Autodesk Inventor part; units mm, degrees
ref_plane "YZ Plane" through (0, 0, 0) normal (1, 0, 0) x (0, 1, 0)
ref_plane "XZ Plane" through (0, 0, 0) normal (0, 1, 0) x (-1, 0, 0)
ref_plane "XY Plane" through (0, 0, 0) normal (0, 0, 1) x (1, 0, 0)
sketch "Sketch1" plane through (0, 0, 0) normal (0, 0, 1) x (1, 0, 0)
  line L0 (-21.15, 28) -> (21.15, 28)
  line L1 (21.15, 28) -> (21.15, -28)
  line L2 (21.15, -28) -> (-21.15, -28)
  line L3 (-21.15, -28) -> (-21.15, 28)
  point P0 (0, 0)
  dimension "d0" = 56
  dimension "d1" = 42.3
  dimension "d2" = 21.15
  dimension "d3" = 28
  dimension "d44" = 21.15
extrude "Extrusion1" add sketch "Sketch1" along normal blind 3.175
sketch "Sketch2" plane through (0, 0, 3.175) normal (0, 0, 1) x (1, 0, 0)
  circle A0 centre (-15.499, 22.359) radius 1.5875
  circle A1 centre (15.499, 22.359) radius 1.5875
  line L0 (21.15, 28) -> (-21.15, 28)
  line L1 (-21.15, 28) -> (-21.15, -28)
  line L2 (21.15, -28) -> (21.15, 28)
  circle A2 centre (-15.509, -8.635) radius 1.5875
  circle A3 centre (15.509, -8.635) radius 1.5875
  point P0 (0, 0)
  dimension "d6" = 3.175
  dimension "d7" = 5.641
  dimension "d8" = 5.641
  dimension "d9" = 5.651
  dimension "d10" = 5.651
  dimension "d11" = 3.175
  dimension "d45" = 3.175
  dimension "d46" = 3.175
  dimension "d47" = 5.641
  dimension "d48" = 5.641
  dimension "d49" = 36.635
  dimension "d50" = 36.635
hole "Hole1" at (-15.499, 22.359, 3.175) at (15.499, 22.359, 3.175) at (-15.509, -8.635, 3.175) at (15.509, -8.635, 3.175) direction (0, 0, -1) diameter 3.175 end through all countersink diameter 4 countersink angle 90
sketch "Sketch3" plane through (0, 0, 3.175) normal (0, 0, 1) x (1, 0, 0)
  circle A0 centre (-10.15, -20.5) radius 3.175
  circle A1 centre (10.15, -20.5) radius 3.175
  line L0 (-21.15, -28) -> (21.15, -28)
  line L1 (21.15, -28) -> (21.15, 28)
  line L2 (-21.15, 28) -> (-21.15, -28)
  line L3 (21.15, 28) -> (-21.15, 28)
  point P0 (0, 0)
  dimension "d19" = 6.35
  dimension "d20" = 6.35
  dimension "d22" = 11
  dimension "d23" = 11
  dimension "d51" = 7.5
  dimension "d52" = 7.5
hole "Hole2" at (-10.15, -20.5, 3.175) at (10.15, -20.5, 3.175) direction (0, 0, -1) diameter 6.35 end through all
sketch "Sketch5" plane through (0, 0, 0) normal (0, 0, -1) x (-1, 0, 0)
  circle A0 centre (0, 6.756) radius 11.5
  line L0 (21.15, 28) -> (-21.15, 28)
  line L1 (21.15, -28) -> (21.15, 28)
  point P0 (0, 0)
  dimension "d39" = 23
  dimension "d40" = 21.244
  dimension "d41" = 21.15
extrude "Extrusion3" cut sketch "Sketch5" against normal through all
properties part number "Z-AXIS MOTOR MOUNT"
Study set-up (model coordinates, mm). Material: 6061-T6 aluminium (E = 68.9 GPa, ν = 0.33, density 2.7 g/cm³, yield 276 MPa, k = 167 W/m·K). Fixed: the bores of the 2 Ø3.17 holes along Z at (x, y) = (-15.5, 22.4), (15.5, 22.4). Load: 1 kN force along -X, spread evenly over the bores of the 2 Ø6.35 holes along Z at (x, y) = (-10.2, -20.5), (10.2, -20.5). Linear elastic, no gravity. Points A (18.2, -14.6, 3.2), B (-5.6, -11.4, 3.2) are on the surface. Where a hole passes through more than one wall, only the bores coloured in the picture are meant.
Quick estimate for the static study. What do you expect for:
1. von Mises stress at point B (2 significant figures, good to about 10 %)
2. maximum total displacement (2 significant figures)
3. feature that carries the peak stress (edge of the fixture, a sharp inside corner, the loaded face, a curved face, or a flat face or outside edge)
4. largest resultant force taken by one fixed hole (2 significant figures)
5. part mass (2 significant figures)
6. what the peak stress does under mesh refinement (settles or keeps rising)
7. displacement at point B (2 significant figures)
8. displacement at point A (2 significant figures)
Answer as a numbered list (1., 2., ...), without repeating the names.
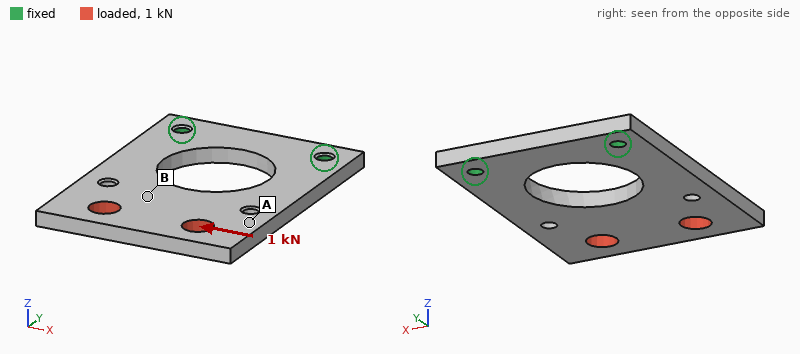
1. 31 MPa
2. 88 µm
3. edge of the fixture
4. 1.3 kN
5. 16 g
6. keeps rising
7. 67 µm
8. 73 µm
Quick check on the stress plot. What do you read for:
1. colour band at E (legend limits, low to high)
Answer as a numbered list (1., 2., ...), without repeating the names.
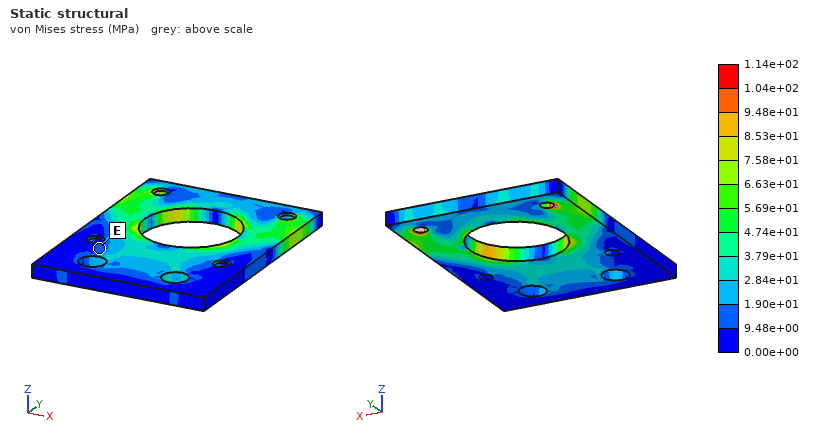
1. 9.48e+00 to 1.90e+01 MPa
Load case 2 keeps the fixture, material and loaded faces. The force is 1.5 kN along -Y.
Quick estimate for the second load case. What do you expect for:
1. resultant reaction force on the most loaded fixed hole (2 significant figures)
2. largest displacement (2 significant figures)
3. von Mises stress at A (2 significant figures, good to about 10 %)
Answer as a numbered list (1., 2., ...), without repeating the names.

1. 750 N
2. 17 µm
3. 15 MPa
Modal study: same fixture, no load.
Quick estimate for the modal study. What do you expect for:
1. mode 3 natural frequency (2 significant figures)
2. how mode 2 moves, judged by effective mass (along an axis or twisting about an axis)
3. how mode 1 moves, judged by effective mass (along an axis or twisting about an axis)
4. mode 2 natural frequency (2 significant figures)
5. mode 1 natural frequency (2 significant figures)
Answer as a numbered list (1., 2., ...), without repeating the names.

1. 5800 Hz
2. twisting about Y
3. along Z
4. 2500 Hz
5. 810 Hz
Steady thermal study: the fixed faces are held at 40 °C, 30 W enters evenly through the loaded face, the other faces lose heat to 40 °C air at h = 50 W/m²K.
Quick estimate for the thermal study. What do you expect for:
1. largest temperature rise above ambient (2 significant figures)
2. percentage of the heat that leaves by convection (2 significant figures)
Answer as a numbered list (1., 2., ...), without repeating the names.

1. 76 K
2. 30 %
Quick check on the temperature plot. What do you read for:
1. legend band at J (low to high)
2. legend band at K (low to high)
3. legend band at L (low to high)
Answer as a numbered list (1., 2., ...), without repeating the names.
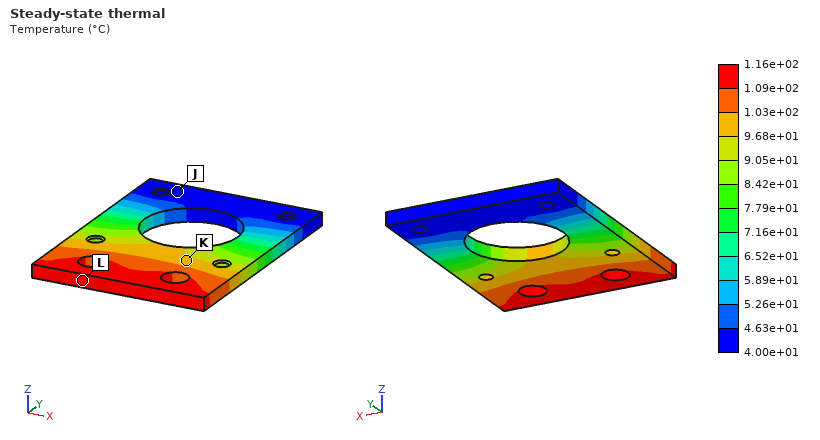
1. 4.00e+01 to 4.63e+01 °C
2. 9.68e+01 to 1.03e+02 °C
3. 1.09e+02 to 1.16e+02 °C
